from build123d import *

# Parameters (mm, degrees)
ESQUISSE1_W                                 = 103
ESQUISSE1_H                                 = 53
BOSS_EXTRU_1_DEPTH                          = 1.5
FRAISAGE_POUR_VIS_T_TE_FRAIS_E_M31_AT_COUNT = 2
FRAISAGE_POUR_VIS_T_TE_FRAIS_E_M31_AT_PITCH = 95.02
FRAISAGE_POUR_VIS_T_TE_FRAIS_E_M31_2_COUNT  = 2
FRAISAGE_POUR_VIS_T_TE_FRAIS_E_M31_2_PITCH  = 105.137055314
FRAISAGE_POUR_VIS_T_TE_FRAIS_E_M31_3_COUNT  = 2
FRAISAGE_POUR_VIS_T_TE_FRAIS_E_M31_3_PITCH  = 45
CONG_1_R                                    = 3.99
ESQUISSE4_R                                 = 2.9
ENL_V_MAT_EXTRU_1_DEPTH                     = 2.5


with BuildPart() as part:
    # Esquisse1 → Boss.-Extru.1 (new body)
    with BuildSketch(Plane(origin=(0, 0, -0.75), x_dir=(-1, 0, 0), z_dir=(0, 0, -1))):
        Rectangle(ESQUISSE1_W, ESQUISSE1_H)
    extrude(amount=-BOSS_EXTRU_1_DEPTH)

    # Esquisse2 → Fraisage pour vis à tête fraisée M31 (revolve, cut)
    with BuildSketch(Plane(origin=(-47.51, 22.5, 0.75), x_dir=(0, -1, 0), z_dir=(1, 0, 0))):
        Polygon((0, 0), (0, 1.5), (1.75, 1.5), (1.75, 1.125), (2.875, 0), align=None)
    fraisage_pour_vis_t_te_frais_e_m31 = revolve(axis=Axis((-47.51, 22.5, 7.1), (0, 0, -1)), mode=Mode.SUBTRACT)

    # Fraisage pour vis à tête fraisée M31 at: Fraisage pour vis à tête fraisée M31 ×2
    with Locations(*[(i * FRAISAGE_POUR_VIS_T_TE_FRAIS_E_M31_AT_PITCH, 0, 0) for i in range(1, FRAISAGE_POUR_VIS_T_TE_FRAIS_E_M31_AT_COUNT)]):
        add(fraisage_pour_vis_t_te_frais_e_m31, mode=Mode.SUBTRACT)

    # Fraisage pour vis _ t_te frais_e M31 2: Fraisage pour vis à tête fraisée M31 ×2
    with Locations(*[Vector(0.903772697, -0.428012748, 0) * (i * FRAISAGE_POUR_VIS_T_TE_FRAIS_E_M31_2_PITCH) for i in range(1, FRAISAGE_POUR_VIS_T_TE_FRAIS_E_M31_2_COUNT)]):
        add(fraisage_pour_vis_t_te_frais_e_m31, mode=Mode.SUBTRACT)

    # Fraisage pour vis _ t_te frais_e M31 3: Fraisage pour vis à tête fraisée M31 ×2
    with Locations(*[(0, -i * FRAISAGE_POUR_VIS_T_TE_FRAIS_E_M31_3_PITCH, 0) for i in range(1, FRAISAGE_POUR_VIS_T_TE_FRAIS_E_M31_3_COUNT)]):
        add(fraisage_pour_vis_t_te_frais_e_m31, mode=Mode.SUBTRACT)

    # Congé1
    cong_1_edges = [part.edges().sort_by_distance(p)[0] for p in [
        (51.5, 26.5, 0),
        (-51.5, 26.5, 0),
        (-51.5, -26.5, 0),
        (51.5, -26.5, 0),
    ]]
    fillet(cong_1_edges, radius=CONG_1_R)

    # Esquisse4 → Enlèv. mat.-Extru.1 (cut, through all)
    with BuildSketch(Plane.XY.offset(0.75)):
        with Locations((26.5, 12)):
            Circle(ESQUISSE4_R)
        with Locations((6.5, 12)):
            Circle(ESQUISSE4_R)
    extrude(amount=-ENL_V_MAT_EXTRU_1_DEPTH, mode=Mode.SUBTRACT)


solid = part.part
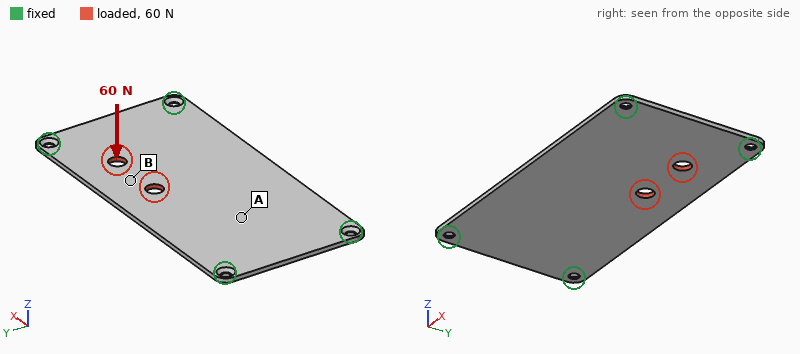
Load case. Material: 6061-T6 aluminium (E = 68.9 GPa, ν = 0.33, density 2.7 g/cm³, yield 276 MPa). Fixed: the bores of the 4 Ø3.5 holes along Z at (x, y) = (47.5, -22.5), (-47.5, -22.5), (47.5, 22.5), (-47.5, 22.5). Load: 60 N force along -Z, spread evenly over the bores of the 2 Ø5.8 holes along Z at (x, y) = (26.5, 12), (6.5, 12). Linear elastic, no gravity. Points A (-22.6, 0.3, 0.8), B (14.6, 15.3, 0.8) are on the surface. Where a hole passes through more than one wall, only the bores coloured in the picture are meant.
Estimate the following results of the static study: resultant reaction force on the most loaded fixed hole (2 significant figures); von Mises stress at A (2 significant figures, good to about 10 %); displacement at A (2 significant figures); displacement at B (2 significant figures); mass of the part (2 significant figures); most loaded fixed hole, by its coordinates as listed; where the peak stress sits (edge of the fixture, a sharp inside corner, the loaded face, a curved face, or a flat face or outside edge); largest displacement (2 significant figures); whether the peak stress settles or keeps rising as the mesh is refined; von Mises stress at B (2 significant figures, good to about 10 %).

98 N
8.6 MPa
0.16 mm
0.33 mm
22 g
(47.5, 22.5)
edge of the fixture
0.39 mm
keeps rising
25 MPa
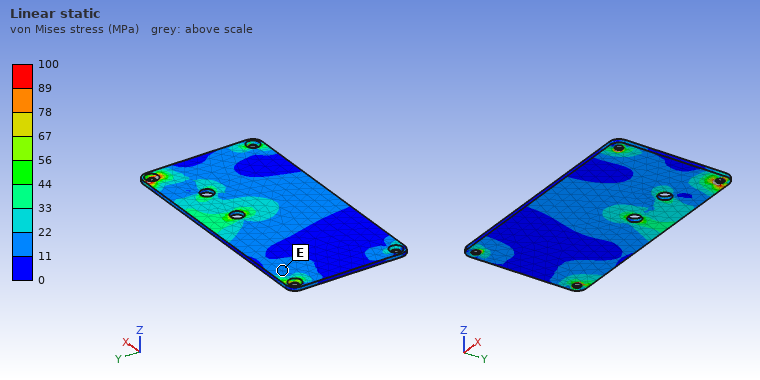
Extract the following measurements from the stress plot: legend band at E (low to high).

11 to 22 MPa
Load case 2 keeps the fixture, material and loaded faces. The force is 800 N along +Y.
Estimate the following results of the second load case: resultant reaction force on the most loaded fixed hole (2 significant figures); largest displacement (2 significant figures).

320 N
20 µm
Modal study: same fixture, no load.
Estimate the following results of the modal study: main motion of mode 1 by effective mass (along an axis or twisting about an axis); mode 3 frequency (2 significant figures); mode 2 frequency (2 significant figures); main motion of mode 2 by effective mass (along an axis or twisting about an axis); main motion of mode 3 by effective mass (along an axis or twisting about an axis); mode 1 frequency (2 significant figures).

along Z
1900 Hz
1300 Hz
twisting about X
twisting about Y
690 Hz
